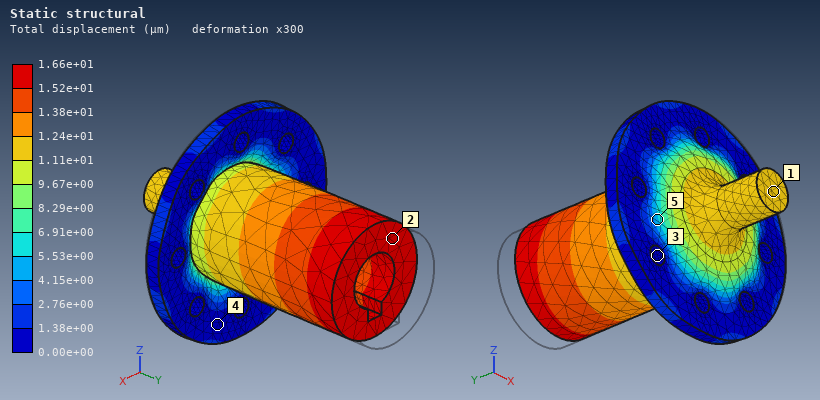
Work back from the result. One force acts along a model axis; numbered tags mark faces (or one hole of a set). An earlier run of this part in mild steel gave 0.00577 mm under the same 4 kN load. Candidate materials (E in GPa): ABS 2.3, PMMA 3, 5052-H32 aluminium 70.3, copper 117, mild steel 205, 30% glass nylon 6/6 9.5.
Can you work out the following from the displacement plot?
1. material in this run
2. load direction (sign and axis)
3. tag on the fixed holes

5052-H32 aluminium
-Y
3
